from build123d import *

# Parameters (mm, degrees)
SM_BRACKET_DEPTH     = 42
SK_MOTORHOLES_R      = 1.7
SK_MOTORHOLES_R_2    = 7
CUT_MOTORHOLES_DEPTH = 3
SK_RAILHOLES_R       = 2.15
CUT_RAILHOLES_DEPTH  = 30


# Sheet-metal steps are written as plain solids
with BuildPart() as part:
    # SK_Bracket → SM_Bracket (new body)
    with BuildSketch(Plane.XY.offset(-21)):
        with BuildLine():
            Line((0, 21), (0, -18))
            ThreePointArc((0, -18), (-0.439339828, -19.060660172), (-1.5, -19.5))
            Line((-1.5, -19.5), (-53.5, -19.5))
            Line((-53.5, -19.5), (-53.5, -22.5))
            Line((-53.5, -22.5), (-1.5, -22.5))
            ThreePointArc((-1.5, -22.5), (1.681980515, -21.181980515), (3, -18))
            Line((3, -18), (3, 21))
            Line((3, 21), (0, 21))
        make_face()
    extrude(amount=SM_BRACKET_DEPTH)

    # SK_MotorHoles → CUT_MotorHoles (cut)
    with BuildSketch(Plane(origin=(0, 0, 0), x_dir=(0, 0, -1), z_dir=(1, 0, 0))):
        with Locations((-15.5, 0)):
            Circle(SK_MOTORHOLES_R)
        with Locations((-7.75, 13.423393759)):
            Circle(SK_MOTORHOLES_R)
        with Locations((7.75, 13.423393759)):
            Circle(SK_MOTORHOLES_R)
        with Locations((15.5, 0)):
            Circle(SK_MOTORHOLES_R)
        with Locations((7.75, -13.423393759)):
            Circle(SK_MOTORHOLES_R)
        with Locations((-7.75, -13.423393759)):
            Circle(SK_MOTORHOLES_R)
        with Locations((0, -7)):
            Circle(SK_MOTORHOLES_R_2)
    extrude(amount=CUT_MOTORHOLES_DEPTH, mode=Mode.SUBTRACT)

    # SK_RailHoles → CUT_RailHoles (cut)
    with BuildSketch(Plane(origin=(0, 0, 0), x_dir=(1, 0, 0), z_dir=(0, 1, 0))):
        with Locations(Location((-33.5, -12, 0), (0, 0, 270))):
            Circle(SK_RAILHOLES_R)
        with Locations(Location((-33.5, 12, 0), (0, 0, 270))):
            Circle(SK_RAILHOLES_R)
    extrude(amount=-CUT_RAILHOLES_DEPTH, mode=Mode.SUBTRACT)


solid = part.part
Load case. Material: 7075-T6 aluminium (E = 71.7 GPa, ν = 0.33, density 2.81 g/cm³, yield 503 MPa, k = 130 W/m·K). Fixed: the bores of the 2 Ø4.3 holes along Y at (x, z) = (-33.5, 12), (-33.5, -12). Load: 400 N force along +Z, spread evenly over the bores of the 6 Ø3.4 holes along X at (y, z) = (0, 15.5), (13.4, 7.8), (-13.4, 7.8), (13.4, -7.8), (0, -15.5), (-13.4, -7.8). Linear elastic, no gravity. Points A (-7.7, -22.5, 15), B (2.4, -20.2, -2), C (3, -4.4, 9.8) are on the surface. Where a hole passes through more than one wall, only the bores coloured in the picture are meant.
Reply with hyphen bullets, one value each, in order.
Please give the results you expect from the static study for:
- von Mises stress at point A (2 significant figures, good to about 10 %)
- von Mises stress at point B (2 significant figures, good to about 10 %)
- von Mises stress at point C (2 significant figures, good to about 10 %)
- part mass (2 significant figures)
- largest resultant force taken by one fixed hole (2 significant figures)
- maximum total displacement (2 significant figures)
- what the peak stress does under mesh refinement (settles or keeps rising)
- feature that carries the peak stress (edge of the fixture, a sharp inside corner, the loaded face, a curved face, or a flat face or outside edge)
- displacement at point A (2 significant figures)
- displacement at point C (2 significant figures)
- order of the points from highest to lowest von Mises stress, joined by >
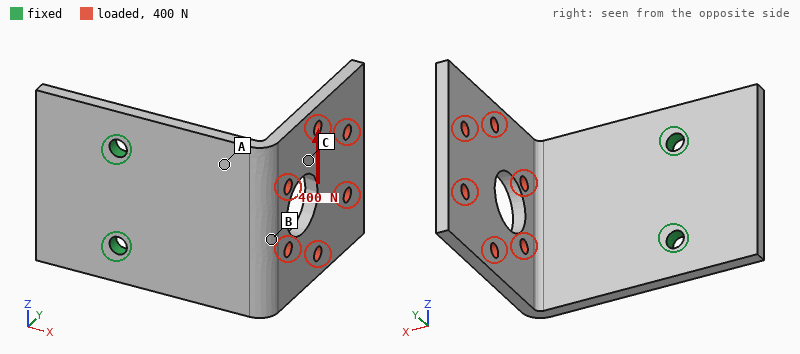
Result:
- 79 MPa
- 46 MPa
- 18 MPa
- 32 g
- 640 N
- 0.85 mm
- keeps rising
- edge of the fixture
- 0.19 mm
- 0.35 mm
- A > B > C
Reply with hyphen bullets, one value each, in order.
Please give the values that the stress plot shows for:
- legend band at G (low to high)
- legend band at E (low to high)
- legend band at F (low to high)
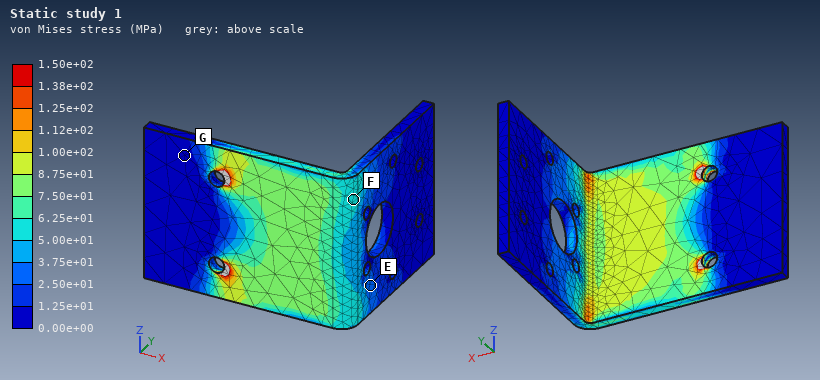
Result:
- 0.00e+00 to 1.25e+01 MPa
- 2.50e+01 to 3.75e+01 MPa
- 5.00e+01 to 6.25e+01 MPa
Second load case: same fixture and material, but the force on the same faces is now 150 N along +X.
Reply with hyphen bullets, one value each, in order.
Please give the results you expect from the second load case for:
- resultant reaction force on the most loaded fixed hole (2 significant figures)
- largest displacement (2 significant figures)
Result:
- 76 N
- 0.93 mm
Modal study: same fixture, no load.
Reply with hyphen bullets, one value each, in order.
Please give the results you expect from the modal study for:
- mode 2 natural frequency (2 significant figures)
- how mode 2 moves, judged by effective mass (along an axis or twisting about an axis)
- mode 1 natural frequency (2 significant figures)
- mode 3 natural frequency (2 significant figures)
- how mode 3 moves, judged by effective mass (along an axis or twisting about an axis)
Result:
- 1000 Hz
- along Z
- 580 Hz
- 1500 Hz
- along Y
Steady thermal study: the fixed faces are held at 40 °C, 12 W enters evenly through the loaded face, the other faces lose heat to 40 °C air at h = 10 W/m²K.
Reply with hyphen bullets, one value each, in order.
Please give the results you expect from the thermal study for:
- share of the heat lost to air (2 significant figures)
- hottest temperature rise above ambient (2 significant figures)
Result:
- 14 %
- 41 K
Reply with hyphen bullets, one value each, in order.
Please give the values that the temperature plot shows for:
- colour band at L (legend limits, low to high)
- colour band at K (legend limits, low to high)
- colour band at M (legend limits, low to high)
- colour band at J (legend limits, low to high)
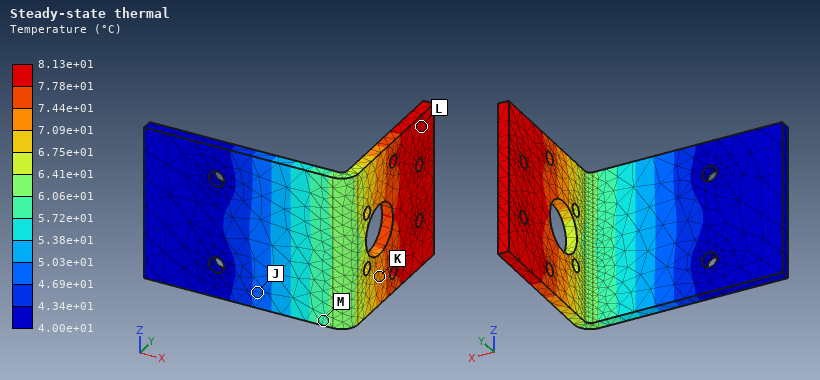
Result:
- 7.78e+01 to 8.13e+01 °C
- 7.09e+01 to 7.44e+01 °C
- 5.72e+01 to 6.06e+01 °C
- 4.69e+01 to 5.03e+01 °C
